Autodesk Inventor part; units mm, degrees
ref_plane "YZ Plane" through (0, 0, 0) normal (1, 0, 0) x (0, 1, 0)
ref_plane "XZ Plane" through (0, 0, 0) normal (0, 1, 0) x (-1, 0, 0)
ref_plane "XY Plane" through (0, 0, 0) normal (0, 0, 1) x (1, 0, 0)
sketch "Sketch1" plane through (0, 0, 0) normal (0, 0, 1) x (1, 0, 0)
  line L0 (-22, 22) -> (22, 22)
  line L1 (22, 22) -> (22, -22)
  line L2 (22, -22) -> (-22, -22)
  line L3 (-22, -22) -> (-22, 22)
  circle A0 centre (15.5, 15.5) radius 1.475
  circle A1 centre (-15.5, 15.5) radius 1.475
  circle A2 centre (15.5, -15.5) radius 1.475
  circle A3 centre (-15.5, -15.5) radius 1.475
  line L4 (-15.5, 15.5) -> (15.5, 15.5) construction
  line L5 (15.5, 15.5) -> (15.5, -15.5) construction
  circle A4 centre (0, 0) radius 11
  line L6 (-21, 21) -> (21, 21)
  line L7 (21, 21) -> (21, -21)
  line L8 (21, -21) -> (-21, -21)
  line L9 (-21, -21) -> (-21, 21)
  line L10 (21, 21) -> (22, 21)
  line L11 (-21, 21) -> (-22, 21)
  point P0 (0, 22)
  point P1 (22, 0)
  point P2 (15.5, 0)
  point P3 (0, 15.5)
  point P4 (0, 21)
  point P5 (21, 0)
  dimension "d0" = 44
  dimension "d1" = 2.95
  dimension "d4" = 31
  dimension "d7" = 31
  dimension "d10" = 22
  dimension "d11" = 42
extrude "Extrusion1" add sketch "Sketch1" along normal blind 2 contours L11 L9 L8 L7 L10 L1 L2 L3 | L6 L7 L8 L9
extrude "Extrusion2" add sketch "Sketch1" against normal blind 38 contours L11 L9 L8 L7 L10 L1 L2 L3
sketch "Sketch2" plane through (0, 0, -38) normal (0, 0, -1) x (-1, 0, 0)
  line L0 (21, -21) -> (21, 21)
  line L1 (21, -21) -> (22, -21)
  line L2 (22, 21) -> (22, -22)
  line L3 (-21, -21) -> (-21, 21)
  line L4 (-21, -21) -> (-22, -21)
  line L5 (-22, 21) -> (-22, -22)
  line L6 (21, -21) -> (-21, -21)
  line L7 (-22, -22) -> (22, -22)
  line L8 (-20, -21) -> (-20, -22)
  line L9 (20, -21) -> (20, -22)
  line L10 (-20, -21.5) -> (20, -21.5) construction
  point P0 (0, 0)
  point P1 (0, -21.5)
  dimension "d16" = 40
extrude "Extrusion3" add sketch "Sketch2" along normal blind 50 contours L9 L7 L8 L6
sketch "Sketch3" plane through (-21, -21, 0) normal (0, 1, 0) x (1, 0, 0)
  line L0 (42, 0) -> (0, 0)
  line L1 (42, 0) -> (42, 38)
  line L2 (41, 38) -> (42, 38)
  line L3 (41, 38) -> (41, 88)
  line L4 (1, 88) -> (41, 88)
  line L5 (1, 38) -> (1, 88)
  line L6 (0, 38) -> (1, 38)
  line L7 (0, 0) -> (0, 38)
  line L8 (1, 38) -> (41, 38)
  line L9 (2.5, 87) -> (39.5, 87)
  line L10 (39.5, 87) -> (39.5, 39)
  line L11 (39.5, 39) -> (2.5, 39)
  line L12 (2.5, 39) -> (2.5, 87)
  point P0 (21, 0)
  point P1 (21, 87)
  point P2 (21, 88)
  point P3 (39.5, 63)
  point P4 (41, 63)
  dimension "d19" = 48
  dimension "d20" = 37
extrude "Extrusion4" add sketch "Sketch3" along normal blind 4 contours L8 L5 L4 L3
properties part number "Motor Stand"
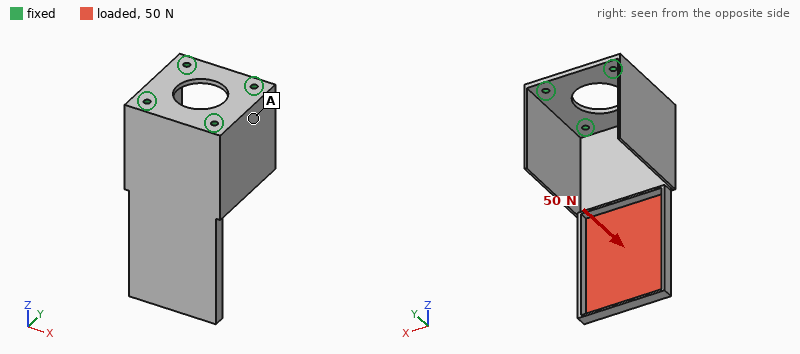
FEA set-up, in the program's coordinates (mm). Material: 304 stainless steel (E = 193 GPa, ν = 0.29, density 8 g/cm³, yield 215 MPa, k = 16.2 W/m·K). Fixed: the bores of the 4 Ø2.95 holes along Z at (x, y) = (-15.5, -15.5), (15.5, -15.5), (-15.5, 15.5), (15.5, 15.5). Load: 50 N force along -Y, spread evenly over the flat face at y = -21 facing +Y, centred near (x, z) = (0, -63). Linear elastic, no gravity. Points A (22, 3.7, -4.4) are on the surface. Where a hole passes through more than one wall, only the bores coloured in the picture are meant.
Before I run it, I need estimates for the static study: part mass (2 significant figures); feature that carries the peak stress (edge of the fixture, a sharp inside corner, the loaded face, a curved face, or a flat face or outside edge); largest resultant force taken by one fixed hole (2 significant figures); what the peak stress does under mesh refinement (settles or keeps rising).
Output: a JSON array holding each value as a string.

["86 g", "a sharp inside corner", "51 N", "keeps rising"]
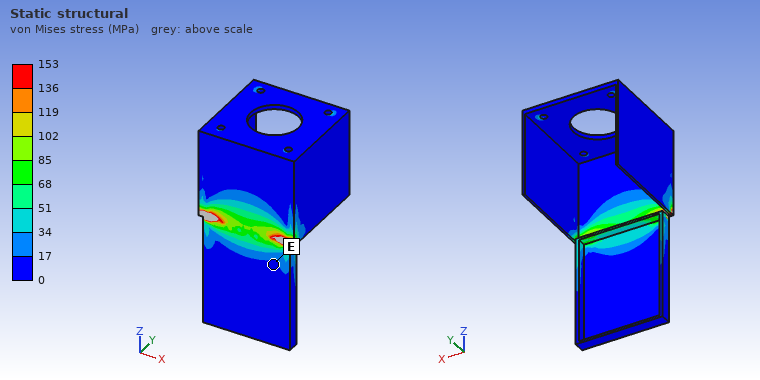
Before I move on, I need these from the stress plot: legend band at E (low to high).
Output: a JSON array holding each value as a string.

["0 to 17 MPa"]
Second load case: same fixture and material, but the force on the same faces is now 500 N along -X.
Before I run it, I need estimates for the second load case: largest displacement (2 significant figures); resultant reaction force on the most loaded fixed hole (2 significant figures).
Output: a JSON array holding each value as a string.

["0.18 mm", "1.0 kN"]
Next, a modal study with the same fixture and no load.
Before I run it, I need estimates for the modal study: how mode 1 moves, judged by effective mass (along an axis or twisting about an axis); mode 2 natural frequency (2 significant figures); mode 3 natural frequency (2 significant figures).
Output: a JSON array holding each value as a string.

["along Y", "890 Hz", "920 Hz"]
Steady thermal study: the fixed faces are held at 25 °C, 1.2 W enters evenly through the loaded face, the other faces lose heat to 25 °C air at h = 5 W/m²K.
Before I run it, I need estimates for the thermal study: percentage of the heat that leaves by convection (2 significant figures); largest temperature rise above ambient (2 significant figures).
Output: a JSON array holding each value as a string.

["69 %", "36 K"]
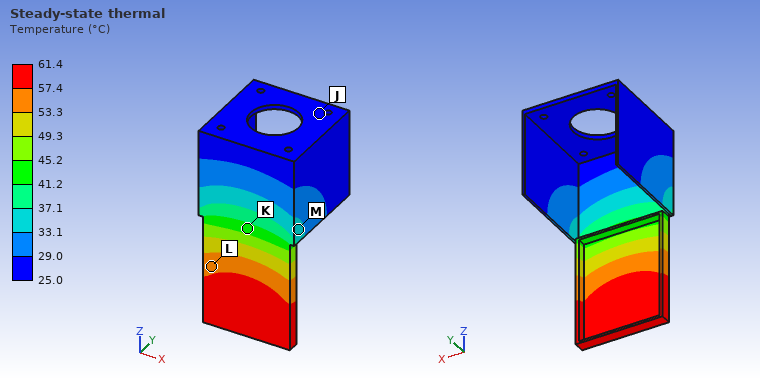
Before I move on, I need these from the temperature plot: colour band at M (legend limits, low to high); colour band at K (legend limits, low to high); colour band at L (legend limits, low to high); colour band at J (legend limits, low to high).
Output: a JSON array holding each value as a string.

["33.1 to 37.1 °C", "41.2 to 45.2 °C", "53.3 to 57.4 °C", "25.0 to 29.0 °C"]
